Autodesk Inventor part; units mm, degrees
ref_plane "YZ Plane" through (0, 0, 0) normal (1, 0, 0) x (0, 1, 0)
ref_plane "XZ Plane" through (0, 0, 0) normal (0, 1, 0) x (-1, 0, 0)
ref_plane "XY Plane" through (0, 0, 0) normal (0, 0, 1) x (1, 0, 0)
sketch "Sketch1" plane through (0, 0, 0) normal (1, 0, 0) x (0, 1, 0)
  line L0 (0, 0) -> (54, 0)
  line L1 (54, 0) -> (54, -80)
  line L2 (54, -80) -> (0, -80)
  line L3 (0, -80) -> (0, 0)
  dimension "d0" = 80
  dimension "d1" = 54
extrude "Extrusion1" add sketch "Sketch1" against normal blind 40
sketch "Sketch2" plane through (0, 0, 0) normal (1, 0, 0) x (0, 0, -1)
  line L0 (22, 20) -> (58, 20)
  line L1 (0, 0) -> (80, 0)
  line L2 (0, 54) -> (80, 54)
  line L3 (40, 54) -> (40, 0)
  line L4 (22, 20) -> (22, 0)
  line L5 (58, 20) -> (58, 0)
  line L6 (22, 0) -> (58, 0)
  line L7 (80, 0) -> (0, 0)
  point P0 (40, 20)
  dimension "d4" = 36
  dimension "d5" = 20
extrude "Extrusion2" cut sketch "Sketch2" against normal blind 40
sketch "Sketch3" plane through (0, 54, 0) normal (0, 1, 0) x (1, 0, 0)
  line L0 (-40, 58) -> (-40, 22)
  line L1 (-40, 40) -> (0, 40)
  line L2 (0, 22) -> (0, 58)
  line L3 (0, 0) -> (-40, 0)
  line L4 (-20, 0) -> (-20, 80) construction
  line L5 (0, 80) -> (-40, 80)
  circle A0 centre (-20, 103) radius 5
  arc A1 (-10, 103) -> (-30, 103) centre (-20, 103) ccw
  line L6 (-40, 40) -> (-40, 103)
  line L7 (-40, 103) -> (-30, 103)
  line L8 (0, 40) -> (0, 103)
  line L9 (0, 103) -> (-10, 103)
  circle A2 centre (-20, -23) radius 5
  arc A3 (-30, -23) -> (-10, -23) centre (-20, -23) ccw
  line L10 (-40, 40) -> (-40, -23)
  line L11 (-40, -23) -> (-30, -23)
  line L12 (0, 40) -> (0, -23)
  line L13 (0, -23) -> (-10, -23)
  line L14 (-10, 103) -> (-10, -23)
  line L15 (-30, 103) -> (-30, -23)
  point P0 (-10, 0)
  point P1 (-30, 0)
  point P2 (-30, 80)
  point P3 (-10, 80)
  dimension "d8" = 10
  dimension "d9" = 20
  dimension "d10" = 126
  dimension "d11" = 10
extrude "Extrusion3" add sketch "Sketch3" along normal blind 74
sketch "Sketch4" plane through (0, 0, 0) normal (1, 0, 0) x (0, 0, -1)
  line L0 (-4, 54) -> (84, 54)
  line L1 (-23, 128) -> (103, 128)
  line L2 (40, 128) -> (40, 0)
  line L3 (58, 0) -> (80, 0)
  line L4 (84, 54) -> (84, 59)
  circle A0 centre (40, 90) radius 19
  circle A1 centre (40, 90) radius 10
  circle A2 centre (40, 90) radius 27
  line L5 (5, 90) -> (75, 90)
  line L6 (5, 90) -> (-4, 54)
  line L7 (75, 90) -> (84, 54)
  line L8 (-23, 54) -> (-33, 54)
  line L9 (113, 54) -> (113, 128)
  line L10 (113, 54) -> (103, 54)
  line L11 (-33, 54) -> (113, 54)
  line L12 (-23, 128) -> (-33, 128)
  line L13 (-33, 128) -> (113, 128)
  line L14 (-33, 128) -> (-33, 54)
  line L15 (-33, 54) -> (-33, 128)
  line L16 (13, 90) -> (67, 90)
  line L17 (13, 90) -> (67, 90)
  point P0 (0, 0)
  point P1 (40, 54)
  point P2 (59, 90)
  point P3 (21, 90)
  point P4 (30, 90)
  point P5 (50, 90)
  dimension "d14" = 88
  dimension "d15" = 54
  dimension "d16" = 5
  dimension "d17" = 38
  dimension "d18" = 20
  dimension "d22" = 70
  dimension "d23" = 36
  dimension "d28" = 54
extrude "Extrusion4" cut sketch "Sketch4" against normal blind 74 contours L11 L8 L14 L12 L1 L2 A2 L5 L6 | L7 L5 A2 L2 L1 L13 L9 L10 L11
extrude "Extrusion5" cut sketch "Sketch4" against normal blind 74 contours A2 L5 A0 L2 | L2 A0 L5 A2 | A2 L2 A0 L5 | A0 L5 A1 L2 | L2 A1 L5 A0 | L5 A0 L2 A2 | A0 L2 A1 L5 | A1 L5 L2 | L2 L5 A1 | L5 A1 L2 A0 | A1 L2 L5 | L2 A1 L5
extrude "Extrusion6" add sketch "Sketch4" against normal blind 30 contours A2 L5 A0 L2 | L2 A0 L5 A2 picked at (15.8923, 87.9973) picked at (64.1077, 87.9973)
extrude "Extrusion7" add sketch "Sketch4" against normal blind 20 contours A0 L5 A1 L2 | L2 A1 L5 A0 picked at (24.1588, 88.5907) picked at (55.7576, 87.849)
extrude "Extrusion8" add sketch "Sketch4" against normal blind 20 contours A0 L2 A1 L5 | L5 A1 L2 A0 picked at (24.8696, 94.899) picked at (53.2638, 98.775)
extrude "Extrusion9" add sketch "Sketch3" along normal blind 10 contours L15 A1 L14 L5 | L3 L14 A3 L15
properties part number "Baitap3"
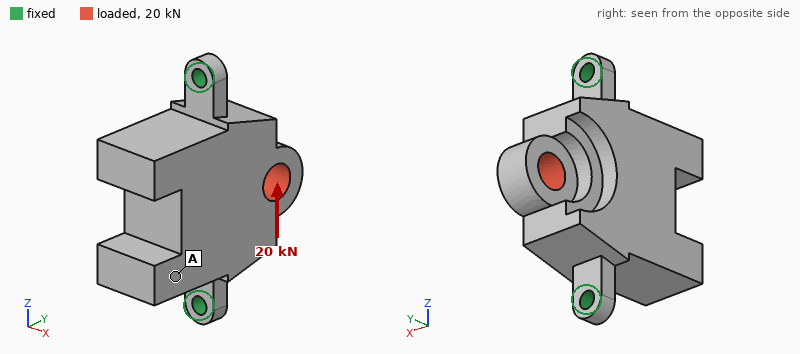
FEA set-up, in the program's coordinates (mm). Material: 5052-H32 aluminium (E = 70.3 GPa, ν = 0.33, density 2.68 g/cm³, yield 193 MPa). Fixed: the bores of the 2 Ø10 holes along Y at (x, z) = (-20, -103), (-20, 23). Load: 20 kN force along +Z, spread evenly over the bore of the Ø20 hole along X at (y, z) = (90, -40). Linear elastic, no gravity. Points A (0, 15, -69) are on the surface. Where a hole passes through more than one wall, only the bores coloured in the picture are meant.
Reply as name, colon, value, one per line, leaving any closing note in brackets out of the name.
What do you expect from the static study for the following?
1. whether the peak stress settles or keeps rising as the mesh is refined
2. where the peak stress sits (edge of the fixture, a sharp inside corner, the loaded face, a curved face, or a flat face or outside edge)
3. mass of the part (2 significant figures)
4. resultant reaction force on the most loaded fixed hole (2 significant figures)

whether the peak stress settles or keeps rising as the mesh is refined: keeps rising
where the peak stress sits: edge of the fixture
mass of the part: 680 g
resultant reaction force on the most loaded fixed hole: 12 kN
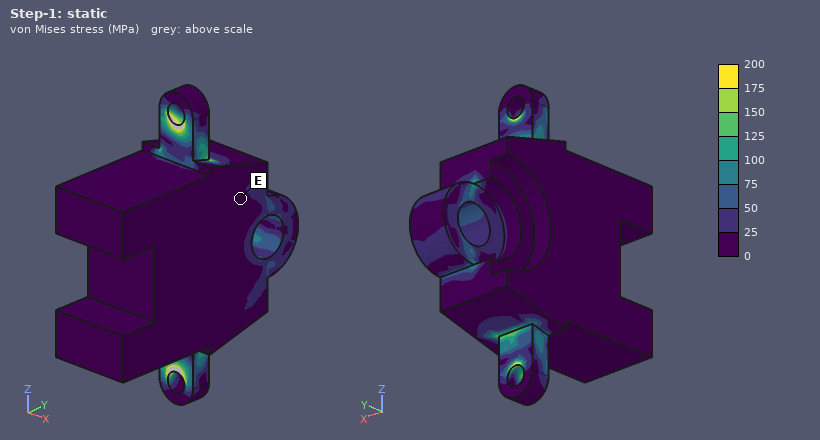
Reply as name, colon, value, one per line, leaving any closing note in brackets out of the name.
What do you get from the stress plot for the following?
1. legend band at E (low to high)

legend band at E: 0 to 25 MPa
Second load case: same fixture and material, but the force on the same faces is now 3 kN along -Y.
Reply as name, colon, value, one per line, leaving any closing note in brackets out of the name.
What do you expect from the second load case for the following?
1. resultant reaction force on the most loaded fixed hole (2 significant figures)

resultant reaction force on the most loaded fixed hole: 1.5 kN
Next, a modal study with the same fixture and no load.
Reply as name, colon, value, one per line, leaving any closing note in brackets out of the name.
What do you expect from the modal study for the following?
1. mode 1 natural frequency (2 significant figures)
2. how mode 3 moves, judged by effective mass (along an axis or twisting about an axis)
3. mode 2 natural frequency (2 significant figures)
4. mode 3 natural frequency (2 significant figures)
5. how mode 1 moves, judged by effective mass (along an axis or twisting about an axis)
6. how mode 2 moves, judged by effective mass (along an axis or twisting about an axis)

mode 1 natural frequency: 780 Hz
how mode 3 moves, judged by effective mass: along X
mode 2 natural frequency: 2500 Hz
mode 3 natural frequency: 3200 Hz
how mode 1 moves, judged by effective mass: along X
how mode 2 moves, judged by effective mass: along Y
